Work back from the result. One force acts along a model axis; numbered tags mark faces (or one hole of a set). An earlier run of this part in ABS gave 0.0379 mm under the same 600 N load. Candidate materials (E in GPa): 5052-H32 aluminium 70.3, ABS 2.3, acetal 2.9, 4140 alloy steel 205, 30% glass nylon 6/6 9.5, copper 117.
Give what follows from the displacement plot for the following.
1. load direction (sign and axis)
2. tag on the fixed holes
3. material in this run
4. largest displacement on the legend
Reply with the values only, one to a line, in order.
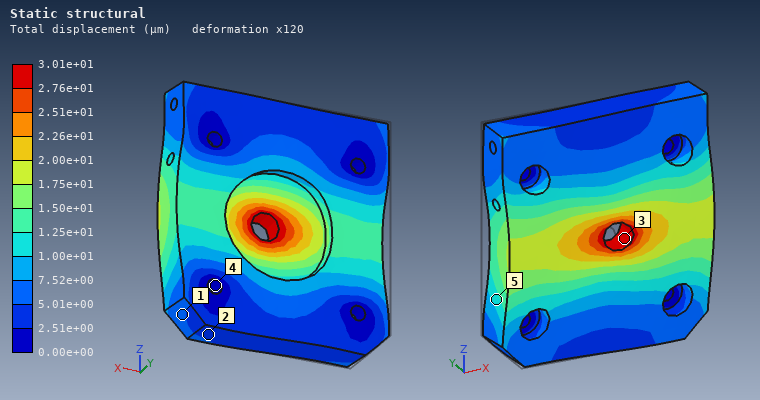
+X
4
acetal
3.01e+01 µm
